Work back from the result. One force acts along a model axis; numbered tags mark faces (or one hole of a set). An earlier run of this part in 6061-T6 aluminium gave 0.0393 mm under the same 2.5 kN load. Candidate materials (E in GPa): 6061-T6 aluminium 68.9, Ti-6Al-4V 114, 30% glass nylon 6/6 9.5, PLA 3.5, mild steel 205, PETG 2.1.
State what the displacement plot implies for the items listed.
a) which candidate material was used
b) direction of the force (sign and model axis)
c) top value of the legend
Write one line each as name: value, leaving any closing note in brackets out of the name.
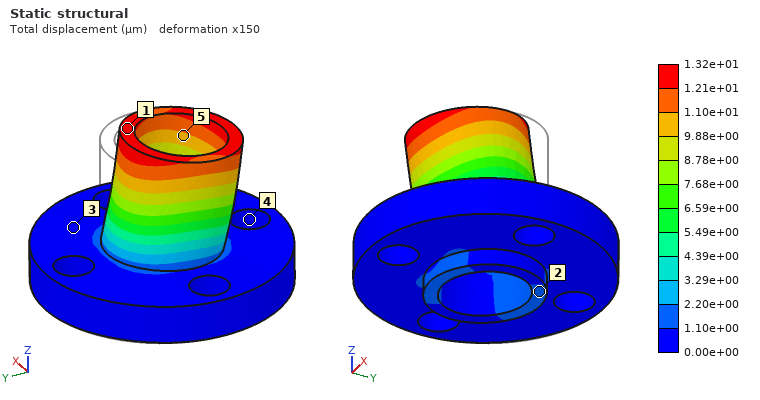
which candidate material was used: mild steel
direction of the force: -Y
top value of the legend: 1.32e+01 µm
